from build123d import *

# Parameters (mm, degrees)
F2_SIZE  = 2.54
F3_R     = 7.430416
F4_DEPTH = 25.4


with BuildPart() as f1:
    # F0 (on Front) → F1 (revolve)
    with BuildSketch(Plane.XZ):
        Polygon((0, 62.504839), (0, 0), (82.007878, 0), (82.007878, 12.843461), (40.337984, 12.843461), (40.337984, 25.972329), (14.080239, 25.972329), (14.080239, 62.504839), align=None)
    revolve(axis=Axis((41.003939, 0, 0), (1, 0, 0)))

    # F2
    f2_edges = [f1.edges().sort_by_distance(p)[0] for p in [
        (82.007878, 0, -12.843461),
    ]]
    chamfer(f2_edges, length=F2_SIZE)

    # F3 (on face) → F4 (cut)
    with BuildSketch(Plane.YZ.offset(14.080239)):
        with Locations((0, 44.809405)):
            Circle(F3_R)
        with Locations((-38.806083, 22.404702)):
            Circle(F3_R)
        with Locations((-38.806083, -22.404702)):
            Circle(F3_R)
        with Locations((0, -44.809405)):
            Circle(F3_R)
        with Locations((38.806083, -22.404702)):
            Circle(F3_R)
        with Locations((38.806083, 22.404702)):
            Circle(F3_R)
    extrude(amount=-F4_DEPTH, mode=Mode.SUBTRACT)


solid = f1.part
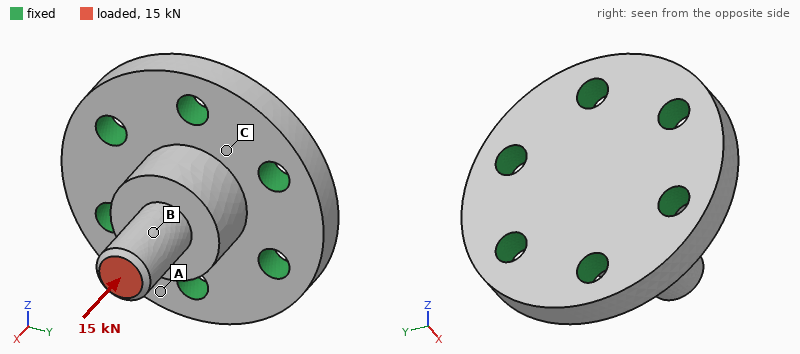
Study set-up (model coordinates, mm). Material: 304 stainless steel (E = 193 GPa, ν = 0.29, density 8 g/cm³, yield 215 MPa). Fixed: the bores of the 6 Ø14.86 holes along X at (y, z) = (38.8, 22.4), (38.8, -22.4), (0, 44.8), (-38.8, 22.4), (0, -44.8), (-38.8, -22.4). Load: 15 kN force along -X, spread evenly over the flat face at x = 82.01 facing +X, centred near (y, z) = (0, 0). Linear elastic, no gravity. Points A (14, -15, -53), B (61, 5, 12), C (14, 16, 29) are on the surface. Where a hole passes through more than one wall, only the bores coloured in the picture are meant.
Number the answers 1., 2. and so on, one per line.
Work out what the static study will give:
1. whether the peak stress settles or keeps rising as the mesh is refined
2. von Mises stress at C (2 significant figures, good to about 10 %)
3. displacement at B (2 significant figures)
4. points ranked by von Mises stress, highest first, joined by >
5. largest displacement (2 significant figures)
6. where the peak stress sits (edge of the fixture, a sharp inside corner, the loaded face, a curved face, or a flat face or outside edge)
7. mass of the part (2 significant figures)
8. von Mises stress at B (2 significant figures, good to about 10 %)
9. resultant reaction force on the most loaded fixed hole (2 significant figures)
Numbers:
1. keeps rising
2. 6.1 MPa
3. 8.1 µm
4. B > C > A
5. 12 µm
6. edge of the fixture
7. 1.9 kg
8. 29 MPa
9. 2.7 kN
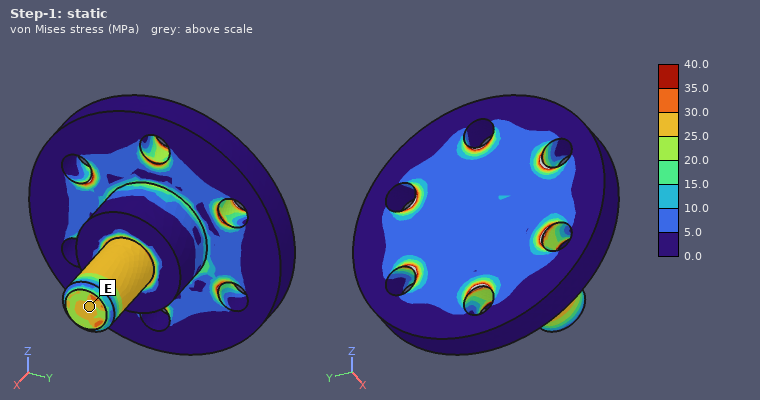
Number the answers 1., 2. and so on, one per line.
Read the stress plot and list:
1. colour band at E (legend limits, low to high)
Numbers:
1. 25.0 to 30.0 MPa
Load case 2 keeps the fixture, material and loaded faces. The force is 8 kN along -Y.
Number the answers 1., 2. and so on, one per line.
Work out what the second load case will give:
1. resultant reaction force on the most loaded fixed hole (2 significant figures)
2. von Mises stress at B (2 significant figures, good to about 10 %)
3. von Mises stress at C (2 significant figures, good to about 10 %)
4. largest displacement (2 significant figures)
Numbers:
1. 5.3 kN
2. 49 MPa
3. 11 MPa
4. 0.10 mm
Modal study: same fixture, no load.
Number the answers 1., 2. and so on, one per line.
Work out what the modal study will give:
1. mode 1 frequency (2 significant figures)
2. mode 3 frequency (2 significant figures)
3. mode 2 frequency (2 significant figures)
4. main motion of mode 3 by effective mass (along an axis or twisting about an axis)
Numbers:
1. 5700 Hz
2. 11 kHz
3. 5700 Hz
4. along X
